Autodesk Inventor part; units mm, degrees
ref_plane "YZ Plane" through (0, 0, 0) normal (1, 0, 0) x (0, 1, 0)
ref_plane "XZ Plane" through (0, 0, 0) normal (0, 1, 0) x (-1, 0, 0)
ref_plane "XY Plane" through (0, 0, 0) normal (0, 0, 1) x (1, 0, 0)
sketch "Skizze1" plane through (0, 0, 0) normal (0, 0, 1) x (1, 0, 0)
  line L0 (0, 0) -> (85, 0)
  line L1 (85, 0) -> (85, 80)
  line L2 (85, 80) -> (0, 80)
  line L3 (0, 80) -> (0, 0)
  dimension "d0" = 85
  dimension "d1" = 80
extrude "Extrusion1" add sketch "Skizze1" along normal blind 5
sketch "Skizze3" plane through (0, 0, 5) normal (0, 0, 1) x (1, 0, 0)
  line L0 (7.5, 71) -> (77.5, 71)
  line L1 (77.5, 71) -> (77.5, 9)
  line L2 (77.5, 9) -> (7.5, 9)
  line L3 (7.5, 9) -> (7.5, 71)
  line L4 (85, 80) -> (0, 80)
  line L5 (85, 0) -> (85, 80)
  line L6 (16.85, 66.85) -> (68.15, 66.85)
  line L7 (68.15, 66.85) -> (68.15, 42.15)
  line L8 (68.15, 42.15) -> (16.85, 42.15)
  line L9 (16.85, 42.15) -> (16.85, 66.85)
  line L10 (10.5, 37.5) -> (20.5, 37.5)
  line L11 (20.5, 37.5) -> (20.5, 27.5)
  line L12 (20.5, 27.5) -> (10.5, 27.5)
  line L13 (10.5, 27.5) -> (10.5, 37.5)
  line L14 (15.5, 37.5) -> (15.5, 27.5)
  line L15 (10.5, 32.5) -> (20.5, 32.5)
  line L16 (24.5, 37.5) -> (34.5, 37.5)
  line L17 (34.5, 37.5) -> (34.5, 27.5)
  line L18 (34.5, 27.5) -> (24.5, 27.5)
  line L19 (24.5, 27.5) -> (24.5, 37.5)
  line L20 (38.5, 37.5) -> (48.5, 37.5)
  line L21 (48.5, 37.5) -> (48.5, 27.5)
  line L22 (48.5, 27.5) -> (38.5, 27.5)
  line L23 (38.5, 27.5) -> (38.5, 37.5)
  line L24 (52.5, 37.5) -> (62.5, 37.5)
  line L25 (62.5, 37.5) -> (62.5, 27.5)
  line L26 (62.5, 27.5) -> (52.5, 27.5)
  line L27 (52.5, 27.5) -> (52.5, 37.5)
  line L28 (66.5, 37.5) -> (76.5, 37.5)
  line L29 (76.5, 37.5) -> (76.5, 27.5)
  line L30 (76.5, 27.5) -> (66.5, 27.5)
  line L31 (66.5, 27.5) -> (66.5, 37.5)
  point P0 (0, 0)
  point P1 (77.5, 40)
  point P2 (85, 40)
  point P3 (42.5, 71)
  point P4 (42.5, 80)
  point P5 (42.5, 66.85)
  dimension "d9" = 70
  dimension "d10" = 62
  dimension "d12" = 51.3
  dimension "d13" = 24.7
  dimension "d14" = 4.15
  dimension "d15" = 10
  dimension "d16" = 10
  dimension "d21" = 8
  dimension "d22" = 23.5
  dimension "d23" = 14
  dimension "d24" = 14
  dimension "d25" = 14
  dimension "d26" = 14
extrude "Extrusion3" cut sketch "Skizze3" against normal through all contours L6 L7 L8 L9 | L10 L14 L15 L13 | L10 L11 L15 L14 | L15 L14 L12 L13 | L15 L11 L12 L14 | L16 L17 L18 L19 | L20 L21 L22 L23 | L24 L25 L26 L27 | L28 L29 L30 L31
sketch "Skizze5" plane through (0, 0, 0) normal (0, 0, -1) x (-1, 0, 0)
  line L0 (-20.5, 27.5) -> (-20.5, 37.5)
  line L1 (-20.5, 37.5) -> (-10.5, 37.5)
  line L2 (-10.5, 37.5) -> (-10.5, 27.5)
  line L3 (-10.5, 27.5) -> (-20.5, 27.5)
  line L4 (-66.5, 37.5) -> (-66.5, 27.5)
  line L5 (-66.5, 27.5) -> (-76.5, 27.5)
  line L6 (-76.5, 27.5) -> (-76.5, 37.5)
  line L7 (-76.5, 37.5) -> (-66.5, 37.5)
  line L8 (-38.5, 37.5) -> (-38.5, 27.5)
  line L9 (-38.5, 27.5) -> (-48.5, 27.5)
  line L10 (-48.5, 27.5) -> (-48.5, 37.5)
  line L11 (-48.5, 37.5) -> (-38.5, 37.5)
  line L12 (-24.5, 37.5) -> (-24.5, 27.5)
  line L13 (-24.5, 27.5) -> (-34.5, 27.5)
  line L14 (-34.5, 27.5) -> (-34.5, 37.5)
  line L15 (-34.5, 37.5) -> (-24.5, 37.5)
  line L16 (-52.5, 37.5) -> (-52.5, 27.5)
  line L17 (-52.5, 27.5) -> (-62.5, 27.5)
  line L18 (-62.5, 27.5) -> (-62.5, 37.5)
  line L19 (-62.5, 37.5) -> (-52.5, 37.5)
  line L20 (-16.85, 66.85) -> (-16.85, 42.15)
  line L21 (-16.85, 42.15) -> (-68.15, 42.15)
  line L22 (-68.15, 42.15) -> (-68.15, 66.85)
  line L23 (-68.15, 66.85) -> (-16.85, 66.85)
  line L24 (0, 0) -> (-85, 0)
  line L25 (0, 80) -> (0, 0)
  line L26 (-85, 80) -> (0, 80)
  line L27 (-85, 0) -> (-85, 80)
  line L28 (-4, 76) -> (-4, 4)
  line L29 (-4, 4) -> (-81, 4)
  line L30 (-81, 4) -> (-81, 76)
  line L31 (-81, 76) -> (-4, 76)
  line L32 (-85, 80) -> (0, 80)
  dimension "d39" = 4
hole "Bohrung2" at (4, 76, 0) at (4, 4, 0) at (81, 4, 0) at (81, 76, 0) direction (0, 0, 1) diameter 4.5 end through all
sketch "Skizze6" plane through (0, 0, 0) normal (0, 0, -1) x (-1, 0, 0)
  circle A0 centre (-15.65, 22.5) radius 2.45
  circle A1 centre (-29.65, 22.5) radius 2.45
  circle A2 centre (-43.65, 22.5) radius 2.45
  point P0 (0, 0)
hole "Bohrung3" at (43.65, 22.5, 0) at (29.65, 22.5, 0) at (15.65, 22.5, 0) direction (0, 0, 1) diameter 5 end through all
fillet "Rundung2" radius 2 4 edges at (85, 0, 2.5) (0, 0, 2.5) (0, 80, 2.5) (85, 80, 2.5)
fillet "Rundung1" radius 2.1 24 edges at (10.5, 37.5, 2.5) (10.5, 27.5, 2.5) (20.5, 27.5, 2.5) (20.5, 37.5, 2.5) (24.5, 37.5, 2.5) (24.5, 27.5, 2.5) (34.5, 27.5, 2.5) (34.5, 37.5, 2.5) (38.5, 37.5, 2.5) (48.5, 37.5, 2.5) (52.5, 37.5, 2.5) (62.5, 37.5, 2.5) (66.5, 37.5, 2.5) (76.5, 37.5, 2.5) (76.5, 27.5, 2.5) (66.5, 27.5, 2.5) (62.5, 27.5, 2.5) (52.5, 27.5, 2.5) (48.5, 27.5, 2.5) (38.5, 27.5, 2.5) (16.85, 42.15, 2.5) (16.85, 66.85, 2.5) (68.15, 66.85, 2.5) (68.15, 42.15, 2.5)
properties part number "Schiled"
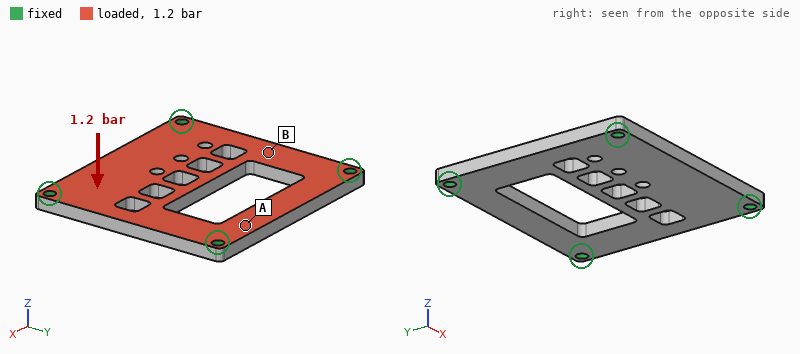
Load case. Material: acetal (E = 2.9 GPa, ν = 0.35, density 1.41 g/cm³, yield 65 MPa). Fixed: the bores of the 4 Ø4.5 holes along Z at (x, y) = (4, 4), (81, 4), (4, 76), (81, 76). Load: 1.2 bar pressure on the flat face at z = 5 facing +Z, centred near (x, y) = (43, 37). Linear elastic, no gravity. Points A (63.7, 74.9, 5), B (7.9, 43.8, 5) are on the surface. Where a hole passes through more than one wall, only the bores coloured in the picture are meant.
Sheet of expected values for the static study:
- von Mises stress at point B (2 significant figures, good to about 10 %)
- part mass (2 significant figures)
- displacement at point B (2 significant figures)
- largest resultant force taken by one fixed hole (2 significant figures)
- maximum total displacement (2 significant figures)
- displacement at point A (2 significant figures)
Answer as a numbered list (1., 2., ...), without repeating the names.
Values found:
1. 8.8 MPa
2. 35 g
3. 0.48 mm
4. 160 N
5. 1.2 mm
6. 0.22 mm
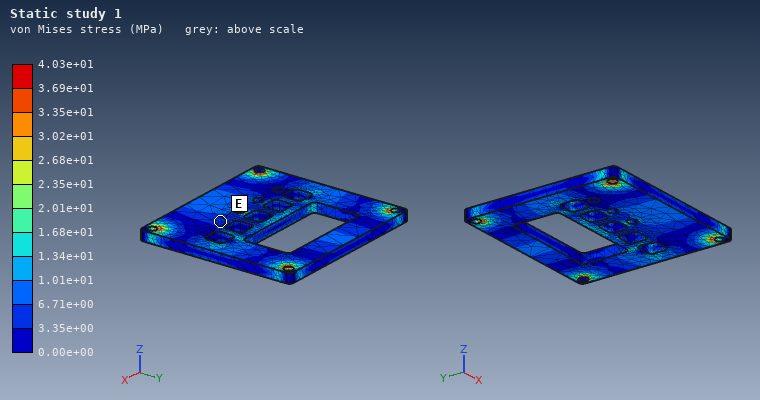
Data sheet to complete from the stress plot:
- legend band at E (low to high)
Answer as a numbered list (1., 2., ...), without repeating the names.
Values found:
1. 3.35e+00 to 6.71e+00 MPa
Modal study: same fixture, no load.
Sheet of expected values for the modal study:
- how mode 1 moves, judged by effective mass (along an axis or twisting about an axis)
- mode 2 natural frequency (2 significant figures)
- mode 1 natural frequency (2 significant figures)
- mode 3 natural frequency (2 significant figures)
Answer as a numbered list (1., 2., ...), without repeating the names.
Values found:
1. along Z
2. 1300 Hz
3. 840 Hz
4. 1400 Hz
